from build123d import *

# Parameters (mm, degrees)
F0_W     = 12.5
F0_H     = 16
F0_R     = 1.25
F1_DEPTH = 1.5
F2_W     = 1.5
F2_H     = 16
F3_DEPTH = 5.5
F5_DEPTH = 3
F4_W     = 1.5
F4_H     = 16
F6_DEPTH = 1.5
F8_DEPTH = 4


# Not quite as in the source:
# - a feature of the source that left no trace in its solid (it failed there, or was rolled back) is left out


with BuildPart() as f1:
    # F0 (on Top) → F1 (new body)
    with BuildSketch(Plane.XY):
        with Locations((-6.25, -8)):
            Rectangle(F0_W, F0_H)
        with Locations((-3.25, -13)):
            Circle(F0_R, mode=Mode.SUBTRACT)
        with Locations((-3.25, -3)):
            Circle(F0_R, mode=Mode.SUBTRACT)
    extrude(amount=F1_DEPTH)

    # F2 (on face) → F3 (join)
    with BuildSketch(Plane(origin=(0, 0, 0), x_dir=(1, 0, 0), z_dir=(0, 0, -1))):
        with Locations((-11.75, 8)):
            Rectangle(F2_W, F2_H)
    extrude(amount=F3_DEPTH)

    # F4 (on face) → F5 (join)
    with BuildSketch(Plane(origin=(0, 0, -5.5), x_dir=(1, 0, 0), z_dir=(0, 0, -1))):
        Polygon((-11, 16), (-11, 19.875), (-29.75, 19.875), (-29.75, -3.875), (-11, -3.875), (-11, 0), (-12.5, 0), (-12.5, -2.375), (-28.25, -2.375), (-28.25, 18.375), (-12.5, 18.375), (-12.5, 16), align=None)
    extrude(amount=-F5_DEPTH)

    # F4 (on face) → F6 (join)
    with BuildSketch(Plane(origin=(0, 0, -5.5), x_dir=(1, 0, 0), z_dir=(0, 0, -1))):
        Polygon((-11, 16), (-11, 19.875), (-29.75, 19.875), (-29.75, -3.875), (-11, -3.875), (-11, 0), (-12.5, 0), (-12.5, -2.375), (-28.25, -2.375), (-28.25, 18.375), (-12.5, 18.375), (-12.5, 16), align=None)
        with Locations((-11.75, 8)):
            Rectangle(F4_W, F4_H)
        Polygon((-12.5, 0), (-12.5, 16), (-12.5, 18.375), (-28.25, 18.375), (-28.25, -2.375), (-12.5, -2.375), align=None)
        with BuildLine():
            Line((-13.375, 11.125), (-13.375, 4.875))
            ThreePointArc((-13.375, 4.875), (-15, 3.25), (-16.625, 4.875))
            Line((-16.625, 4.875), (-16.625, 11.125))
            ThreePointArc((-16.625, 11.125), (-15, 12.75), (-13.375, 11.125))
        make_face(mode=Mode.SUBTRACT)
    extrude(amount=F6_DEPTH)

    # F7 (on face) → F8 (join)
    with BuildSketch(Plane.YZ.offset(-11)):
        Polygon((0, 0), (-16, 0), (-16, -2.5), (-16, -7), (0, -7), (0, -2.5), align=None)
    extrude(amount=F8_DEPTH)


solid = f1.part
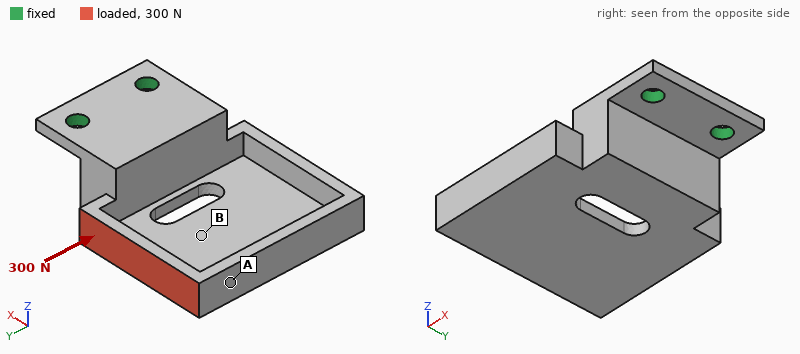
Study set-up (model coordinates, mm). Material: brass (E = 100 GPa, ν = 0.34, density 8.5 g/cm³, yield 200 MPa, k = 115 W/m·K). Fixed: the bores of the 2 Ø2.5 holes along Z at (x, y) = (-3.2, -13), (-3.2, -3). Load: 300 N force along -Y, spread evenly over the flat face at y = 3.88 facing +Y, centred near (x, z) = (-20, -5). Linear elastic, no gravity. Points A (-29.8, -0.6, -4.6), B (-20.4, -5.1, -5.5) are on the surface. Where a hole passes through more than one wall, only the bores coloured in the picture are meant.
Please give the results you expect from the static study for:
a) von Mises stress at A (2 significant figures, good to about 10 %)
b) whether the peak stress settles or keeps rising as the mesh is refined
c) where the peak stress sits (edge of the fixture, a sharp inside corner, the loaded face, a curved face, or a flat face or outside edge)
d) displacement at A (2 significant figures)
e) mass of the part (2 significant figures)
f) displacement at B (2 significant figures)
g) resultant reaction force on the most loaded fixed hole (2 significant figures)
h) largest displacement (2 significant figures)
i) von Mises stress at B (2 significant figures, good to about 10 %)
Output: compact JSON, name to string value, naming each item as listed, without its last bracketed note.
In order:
{"von Mises stress at A": "12 MPa", "whether the peak stress settles or keeps rising as the mesh is refined": "keeps rising", "where the peak stress sits": "edge of the fixture", "displacement at A": "50 µm", "mass of the part": "15 g", "displacement at B": "30 µm", "resultant reaction force on the most loaded fixed hole": "500 N", "largest displacement": "59 µm", "von Mises stress at B": "34 MPa"}
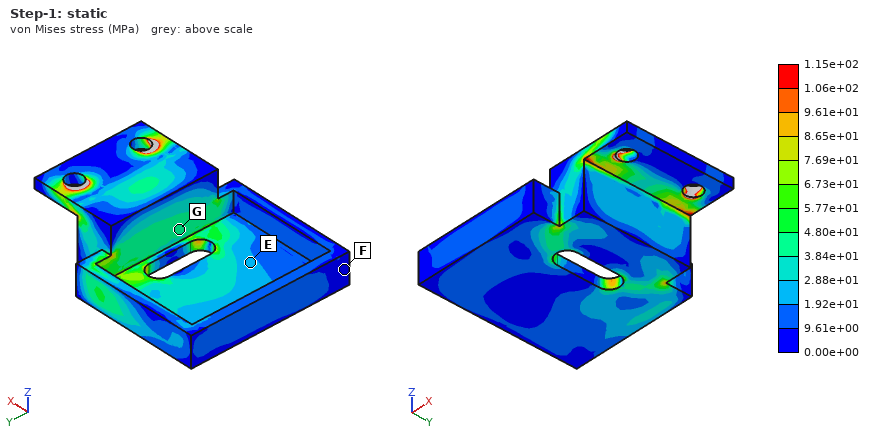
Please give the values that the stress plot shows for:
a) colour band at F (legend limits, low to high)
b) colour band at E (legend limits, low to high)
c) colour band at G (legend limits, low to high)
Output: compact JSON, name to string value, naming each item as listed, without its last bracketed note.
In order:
{"colour band at F": "0.00e+00 to 9.61e+00 MPa", "colour band at E": "1.92e+01 to 2.88e+01 MPa", "colour band at G": "3.84e+01 to 4.80e+01 MPa"}
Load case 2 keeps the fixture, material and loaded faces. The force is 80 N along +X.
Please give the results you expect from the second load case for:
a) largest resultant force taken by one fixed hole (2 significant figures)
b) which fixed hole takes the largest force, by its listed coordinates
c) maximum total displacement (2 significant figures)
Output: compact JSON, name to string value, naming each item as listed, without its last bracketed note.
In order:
{"largest resultant force taken by one fixed hole": "130 N", "which fixed hole takes the largest force, by its listed coordinates": "(-3.2, -3)", "maximum total displacement": "88 µm"}
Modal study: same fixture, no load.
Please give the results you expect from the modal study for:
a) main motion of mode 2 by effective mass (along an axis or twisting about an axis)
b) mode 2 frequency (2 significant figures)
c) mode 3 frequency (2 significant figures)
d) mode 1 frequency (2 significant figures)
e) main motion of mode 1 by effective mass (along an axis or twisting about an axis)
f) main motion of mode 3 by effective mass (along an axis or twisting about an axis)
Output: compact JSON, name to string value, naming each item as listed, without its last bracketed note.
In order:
{"main motion of mode 2 by effective mass": "twisting about X", "mode 2 frequency": "3800 Hz", "mode 3 frequency": "4900 Hz", "mode 1 frequency": "1000 Hz", "main motion of mode 1 by effective mass": "along Z", "main motion of mode 3 by effective mass": "along Y"}
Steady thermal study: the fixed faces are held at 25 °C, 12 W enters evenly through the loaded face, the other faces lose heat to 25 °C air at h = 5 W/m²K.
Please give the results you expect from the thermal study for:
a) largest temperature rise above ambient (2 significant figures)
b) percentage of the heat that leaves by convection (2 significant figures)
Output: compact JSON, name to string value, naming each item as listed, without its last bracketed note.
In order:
{"largest temperature rise above ambient": "79 K", "percentage of the heat that leaves by convection": "3.1 %"}
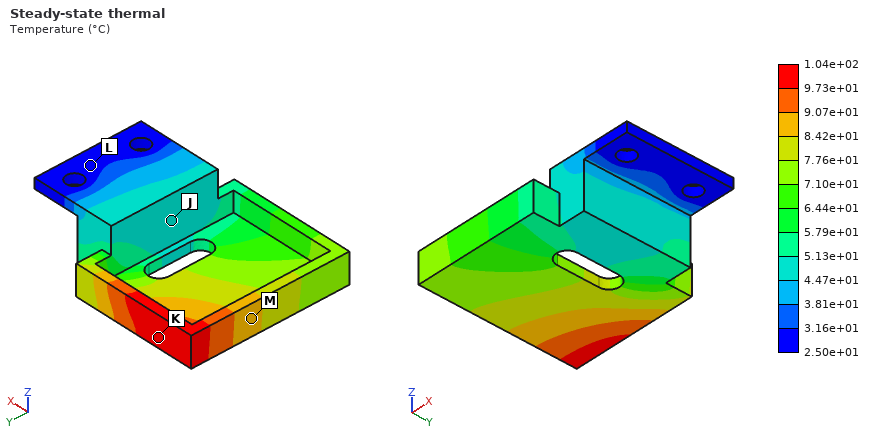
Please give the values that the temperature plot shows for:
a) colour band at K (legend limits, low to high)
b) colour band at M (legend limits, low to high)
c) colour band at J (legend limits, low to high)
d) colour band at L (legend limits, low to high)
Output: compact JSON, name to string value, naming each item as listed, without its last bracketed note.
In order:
{"colour band at K": "9.73e+01 to 1.04e+02 °C", "colour band at M": "8.42e+01 to 9.07e+01 °C", "colour band at J": "4.47e+01 to 5.13e+01 °C", "colour band at L": "2.50e+01 to 3.16e+01 °C"}
